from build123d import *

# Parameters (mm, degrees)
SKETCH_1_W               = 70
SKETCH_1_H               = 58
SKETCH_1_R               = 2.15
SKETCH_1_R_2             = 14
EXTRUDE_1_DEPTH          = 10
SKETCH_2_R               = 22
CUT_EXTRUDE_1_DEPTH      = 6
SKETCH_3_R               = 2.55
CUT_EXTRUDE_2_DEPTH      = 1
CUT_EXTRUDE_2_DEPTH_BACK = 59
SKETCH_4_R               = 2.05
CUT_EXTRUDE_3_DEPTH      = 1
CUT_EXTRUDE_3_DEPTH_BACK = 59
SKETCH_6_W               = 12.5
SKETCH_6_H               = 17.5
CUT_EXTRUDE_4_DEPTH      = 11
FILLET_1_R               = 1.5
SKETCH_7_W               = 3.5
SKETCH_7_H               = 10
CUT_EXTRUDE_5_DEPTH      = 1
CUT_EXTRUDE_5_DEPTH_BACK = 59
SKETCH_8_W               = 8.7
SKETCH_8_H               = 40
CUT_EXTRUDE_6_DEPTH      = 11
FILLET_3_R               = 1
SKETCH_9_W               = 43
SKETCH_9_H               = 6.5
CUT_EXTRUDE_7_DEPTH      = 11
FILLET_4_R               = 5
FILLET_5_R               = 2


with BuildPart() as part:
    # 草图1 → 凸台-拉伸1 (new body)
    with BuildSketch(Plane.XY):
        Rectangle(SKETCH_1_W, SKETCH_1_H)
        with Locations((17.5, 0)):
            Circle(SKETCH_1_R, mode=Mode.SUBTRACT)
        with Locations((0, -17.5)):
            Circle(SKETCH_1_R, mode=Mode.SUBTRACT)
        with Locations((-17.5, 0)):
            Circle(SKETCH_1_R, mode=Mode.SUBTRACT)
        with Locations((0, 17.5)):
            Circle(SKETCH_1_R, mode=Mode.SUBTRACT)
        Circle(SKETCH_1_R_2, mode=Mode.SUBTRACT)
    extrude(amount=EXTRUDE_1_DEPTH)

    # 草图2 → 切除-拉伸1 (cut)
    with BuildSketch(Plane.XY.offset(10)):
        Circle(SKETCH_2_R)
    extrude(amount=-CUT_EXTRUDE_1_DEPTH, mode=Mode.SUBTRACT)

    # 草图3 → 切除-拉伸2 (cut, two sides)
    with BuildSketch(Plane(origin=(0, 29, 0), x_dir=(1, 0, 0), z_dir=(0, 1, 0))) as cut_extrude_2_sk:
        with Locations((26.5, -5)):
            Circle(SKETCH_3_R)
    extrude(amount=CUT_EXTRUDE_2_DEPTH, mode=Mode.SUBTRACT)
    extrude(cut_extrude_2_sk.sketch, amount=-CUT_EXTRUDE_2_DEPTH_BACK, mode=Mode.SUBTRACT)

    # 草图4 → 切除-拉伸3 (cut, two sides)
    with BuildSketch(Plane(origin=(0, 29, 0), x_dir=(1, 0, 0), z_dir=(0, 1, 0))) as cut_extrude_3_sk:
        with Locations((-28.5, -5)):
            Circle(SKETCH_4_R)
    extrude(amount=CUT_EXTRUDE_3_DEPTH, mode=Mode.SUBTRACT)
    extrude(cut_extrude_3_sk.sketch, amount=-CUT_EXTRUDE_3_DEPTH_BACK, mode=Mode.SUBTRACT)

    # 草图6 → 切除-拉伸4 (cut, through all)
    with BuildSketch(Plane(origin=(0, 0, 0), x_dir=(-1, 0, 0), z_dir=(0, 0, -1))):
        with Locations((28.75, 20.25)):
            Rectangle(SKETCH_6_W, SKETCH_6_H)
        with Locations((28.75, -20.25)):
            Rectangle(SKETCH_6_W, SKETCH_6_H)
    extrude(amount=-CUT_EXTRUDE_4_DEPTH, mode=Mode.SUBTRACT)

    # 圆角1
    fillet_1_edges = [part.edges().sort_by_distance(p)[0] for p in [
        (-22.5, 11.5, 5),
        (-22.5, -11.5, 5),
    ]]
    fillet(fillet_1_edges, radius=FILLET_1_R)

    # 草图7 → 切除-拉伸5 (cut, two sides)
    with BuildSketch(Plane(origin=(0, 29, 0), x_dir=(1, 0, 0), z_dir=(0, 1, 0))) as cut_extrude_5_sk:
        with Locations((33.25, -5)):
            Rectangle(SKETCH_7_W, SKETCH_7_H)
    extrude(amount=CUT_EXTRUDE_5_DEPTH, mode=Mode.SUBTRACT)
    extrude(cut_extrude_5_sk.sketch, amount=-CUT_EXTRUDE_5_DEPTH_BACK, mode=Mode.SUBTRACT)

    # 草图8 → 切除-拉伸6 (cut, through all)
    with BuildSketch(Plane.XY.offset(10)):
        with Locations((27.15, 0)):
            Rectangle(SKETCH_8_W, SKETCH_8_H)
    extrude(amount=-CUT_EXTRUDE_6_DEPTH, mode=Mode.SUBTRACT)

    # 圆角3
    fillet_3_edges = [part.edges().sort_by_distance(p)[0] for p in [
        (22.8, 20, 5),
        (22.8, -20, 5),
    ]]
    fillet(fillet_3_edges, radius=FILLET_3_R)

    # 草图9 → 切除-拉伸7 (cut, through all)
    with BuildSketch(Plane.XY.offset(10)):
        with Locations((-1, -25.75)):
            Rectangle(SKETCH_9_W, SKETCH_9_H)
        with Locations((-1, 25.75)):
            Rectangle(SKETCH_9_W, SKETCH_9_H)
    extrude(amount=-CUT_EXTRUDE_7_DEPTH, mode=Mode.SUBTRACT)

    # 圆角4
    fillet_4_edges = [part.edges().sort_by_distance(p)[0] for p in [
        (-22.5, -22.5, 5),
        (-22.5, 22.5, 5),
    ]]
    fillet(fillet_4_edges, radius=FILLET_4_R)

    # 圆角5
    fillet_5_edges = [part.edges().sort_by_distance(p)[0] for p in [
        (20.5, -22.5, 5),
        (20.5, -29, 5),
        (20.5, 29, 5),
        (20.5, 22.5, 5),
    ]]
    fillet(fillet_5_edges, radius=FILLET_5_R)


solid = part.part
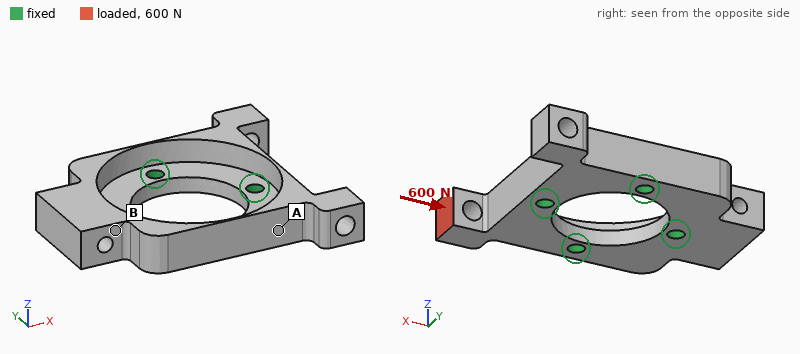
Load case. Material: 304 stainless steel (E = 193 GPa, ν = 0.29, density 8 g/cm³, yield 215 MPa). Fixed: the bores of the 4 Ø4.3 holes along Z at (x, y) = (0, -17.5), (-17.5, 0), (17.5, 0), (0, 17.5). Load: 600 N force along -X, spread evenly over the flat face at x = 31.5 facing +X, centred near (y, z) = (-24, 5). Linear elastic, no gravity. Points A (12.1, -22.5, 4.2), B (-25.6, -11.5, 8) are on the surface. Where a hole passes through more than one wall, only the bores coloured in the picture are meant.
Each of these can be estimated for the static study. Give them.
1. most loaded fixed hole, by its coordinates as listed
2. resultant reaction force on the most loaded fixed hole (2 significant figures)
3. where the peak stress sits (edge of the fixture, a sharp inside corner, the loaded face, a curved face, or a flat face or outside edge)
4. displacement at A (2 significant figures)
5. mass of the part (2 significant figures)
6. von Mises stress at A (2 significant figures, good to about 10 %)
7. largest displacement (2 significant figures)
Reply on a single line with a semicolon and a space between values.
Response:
(0, -17.5); 670 N; a curved face; 3.7 µm; 100 g; 30 MPa; 16 µm
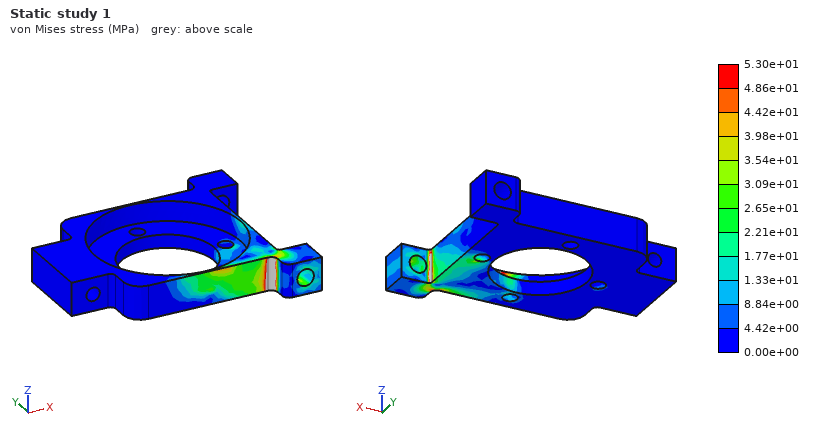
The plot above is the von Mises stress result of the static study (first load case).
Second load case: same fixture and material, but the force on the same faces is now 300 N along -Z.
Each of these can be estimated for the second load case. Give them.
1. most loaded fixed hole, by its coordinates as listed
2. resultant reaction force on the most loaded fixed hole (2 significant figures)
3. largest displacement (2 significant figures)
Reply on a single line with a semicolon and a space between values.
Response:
(17.5, 0); 300 N; 69 µm
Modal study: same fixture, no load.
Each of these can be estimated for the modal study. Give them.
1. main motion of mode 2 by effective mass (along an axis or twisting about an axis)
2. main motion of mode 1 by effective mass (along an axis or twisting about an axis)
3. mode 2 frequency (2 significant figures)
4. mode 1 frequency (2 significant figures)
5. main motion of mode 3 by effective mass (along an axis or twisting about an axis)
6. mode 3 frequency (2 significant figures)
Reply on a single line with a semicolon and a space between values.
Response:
along Z; twisting about X; 5400 Hz; 4300 Hz; along Z; 8900 Hz
